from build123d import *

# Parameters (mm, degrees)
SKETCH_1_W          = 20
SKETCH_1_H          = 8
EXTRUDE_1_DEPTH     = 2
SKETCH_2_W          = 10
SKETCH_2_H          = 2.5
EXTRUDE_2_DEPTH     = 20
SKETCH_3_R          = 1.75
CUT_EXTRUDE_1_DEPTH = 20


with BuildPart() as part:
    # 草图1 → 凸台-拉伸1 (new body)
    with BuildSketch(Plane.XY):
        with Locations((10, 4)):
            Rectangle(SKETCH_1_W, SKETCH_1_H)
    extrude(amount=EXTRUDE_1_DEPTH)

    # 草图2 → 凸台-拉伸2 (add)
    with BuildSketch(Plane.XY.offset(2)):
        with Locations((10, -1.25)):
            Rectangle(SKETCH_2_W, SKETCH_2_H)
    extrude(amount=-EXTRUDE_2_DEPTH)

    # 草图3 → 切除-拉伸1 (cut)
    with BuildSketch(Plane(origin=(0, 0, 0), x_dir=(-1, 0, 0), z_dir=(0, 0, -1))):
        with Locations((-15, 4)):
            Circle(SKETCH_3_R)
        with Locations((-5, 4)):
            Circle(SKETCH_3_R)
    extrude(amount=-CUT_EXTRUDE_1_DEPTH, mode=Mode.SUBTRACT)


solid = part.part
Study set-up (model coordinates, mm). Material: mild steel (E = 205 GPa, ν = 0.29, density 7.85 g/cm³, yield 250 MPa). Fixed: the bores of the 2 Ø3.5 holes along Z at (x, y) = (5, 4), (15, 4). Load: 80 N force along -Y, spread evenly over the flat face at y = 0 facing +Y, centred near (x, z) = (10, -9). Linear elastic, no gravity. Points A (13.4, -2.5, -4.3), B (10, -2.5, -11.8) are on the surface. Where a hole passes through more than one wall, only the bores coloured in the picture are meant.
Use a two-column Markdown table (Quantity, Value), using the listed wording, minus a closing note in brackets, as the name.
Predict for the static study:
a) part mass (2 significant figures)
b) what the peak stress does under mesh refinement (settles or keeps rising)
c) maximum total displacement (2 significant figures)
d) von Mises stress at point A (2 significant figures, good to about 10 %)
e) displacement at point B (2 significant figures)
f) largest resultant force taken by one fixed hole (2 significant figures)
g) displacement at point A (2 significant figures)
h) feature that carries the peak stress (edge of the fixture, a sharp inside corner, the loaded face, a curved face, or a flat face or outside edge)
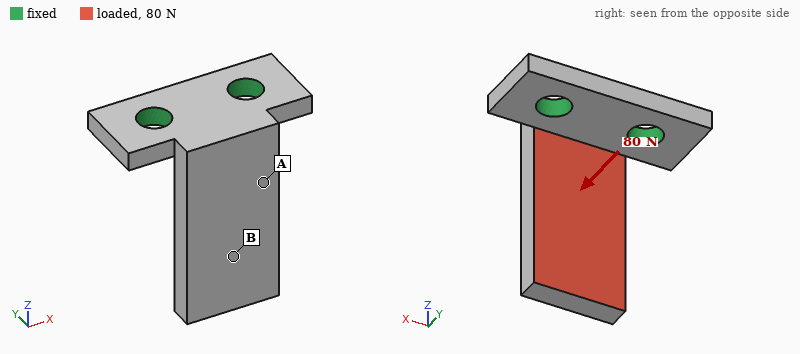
| Quantity | Value |
|---|---|
| part mass | 6.1 g |
| what the peak stress does under mesh refinement | keeps rising |
| maximum total displacement | 60 µm |
| von Mises stress at point A | 40 MPa |
| displacement at point B | 38 µm |
| largest resultant force taken by one fixed hole | 44 N |
| displacement at point A | 15 µm |
| feature that carries the peak stress | a sharp inside corner |
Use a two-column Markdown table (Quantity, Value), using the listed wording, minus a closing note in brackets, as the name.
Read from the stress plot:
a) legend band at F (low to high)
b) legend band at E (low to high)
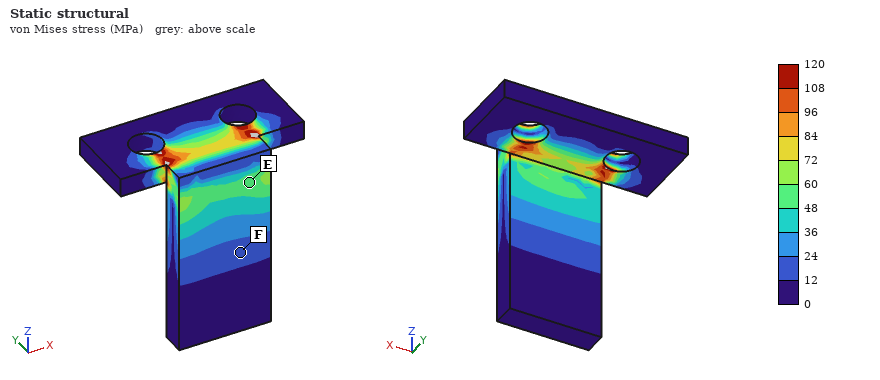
| Quantity | Value |
|---|---|
| legend band at F | 12 to 24 MPa |
| legend band at E | 48 to 60 MPa |
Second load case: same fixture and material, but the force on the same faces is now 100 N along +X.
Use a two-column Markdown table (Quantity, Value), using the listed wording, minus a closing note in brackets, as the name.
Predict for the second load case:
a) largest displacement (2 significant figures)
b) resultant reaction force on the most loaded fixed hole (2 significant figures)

| Quantity | Value |
|---|---|
| largest displacement | 12 µm |
| resultant reaction force on the most loaded fixed hole | 120 N |
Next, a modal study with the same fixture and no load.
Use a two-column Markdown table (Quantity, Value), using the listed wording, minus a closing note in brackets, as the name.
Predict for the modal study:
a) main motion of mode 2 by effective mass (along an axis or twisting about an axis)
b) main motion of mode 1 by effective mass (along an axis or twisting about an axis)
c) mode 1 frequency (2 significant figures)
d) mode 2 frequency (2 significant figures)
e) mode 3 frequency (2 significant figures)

| Quantity | Value |
|---|---|
| main motion of mode 2 by effective mass | along X |
| main motion of mode 1 by effective mass | along Y |
| mode 1 frequency | 3800 Hz |
| mode 2 frequency | 9900 Hz |
| mode 3 frequency | 20 kHz |
